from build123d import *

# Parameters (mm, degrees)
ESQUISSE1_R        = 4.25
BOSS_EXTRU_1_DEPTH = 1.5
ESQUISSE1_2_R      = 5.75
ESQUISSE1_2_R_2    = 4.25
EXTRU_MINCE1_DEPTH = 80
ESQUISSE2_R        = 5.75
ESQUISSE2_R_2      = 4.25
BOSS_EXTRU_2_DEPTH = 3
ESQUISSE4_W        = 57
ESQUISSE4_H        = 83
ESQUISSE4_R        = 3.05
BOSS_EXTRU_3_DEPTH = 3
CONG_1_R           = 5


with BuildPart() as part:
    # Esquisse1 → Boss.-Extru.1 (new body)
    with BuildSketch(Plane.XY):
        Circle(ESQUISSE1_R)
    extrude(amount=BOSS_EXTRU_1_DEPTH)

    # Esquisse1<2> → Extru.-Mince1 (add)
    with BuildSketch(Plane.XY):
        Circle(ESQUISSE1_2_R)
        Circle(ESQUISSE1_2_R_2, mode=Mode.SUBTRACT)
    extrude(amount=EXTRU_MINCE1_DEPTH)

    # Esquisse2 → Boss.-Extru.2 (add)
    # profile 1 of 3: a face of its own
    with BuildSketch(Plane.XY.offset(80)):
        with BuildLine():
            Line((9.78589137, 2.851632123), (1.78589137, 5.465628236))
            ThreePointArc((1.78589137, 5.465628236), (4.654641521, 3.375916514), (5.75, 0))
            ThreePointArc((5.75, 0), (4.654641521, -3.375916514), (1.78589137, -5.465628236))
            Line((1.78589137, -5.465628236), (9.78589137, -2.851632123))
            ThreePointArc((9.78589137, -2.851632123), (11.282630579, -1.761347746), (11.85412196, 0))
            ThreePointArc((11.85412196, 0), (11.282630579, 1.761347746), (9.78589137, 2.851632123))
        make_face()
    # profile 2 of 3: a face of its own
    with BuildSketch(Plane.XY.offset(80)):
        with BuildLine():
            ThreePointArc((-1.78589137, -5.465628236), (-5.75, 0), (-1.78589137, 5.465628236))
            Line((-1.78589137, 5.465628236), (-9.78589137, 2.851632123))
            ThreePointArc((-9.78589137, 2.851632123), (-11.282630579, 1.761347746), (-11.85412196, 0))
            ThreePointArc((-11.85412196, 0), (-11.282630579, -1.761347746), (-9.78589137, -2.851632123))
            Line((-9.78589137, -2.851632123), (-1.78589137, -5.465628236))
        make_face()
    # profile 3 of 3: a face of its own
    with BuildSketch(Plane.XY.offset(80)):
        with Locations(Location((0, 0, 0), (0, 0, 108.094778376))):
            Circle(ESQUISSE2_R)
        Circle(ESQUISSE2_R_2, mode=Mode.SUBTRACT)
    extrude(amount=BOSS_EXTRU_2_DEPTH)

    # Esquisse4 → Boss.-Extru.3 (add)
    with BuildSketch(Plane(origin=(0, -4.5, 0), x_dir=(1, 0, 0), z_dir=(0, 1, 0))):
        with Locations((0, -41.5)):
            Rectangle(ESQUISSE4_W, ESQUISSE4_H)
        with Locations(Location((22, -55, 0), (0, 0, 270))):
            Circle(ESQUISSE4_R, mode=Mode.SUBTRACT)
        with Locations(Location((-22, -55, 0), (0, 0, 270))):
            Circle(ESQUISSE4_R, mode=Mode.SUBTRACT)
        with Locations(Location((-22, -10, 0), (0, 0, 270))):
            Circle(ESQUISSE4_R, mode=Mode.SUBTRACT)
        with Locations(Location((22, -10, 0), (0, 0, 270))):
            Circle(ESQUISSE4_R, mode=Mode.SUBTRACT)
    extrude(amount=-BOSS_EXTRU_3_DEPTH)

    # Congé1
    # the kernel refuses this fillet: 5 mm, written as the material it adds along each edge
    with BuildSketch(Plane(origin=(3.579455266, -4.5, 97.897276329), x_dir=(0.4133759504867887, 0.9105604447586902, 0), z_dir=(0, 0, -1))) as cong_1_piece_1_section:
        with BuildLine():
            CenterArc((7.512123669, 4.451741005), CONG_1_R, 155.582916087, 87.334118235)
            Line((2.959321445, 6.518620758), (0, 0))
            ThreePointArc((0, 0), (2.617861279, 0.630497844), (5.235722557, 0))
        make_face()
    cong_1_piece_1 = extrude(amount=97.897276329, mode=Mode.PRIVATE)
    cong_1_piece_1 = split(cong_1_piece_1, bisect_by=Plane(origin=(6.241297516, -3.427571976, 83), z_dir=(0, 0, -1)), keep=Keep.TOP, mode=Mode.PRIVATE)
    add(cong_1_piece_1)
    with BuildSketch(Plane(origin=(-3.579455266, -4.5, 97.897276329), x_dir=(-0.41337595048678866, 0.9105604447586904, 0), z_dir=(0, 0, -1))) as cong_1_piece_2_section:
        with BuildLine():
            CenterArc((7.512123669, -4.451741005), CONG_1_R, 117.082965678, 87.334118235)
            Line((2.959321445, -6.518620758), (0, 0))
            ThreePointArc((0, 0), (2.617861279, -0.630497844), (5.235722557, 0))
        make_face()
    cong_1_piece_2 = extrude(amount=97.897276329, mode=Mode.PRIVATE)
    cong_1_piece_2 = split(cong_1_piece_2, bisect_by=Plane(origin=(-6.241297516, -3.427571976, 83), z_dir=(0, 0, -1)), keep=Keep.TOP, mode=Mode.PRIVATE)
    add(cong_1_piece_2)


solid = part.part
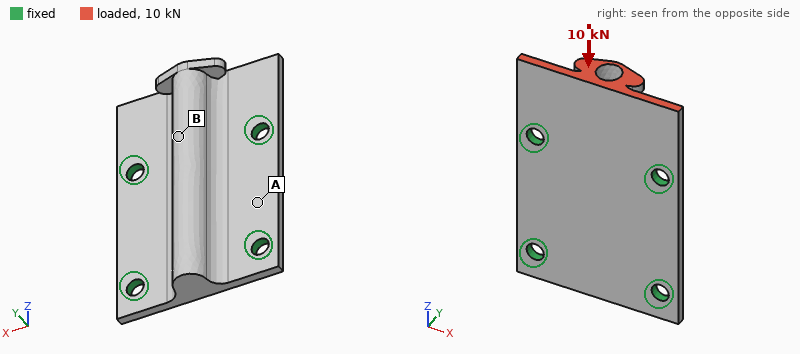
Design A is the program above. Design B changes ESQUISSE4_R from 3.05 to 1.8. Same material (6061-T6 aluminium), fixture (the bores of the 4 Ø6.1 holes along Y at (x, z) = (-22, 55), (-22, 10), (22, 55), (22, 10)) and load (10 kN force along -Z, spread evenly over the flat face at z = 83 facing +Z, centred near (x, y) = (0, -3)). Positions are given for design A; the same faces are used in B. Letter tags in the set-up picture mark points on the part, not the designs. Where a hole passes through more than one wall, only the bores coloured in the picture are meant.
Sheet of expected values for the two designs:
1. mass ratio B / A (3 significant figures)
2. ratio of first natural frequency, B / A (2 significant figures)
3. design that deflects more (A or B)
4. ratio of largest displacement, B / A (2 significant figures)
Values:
1.01
0.88
B
1.1
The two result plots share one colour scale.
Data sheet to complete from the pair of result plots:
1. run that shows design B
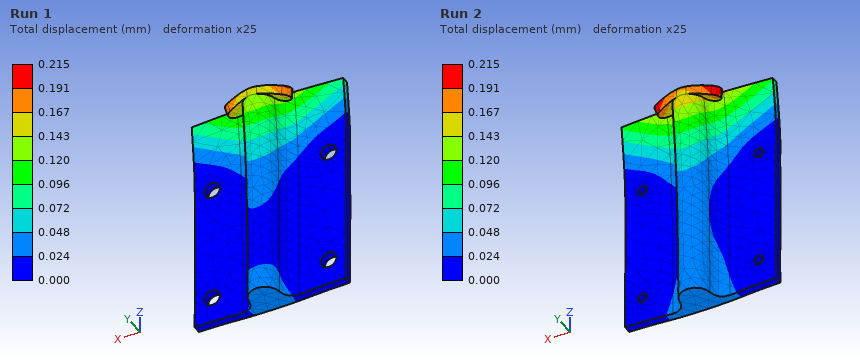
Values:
Run 2
